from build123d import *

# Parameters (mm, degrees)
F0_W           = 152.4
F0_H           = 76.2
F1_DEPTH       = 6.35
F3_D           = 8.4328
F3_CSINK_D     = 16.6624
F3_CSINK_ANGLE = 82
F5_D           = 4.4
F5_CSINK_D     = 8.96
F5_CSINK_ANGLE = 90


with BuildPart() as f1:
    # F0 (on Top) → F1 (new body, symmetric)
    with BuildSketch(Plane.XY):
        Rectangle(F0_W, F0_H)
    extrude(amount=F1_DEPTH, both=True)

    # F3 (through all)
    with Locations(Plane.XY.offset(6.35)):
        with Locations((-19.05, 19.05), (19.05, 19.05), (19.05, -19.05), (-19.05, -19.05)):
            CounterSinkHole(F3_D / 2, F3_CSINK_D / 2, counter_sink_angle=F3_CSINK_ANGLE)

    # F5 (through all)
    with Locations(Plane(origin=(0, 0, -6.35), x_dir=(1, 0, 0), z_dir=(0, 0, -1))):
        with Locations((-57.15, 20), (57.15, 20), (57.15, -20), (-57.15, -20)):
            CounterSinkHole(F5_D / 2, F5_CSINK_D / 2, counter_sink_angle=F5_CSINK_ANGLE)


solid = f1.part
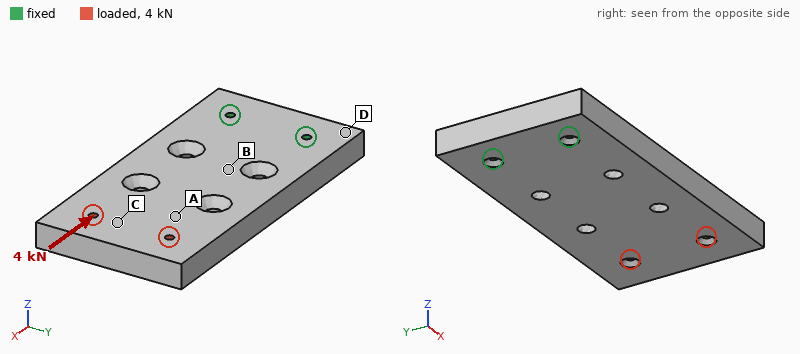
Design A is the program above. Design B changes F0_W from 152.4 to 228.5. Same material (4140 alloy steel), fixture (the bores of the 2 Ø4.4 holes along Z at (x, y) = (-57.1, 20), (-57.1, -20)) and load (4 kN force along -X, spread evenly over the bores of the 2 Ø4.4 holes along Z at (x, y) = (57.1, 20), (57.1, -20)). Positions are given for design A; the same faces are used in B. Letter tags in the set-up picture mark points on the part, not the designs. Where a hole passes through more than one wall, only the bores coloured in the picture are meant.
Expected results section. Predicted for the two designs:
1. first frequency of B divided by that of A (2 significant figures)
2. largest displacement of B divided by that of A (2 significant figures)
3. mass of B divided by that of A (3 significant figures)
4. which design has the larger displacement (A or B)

0.61
1.5
1.52
B
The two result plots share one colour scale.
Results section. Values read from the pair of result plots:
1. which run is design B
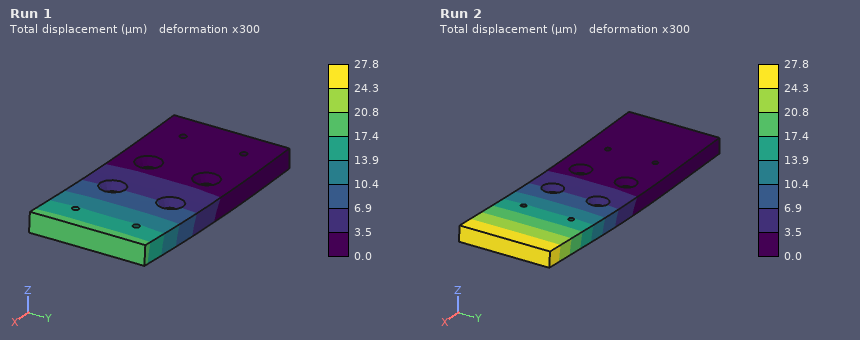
Run 2
